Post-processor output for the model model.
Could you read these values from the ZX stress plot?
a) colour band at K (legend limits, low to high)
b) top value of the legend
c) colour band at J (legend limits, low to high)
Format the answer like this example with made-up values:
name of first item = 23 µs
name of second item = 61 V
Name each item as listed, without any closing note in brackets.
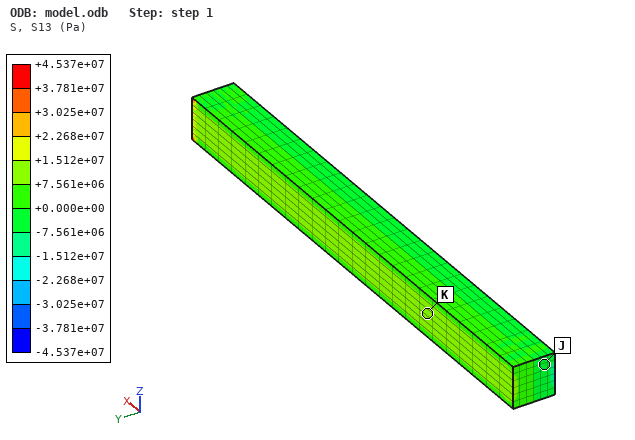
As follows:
colour band at K = +7.561e+06 to +1.512e+07 Pa
top value of the legend = +4.537e+07 Pa
colour band at J = -7.561e+06 to +0.000e+00 Pa
